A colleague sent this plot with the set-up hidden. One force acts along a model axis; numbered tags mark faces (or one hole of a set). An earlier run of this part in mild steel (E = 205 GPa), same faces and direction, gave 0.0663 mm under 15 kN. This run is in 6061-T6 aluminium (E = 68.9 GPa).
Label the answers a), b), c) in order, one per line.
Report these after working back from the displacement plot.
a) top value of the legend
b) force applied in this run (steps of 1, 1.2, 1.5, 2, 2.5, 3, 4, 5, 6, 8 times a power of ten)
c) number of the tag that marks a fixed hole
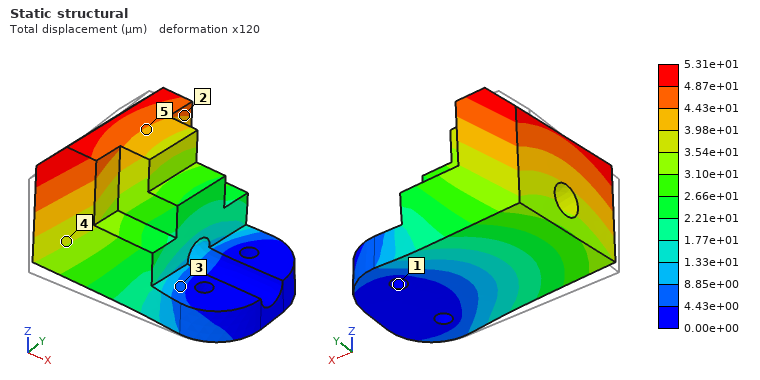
a) 5.31e+01 µm
b) 4 kN
c) 1
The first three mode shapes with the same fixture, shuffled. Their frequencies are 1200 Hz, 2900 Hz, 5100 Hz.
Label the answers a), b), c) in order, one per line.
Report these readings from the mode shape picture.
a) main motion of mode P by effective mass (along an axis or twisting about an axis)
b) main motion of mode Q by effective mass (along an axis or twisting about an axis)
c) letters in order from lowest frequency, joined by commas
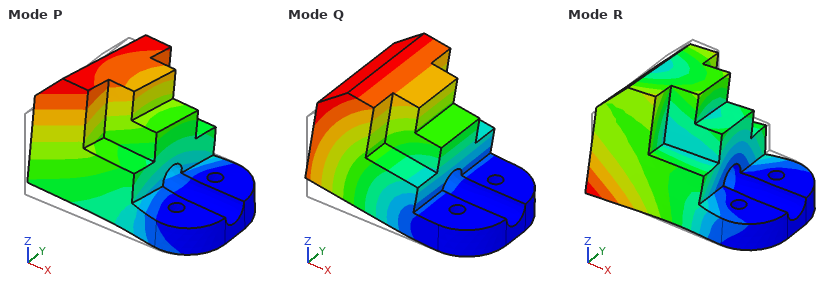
a) along Y
b) along Z
c) Q, P, R
